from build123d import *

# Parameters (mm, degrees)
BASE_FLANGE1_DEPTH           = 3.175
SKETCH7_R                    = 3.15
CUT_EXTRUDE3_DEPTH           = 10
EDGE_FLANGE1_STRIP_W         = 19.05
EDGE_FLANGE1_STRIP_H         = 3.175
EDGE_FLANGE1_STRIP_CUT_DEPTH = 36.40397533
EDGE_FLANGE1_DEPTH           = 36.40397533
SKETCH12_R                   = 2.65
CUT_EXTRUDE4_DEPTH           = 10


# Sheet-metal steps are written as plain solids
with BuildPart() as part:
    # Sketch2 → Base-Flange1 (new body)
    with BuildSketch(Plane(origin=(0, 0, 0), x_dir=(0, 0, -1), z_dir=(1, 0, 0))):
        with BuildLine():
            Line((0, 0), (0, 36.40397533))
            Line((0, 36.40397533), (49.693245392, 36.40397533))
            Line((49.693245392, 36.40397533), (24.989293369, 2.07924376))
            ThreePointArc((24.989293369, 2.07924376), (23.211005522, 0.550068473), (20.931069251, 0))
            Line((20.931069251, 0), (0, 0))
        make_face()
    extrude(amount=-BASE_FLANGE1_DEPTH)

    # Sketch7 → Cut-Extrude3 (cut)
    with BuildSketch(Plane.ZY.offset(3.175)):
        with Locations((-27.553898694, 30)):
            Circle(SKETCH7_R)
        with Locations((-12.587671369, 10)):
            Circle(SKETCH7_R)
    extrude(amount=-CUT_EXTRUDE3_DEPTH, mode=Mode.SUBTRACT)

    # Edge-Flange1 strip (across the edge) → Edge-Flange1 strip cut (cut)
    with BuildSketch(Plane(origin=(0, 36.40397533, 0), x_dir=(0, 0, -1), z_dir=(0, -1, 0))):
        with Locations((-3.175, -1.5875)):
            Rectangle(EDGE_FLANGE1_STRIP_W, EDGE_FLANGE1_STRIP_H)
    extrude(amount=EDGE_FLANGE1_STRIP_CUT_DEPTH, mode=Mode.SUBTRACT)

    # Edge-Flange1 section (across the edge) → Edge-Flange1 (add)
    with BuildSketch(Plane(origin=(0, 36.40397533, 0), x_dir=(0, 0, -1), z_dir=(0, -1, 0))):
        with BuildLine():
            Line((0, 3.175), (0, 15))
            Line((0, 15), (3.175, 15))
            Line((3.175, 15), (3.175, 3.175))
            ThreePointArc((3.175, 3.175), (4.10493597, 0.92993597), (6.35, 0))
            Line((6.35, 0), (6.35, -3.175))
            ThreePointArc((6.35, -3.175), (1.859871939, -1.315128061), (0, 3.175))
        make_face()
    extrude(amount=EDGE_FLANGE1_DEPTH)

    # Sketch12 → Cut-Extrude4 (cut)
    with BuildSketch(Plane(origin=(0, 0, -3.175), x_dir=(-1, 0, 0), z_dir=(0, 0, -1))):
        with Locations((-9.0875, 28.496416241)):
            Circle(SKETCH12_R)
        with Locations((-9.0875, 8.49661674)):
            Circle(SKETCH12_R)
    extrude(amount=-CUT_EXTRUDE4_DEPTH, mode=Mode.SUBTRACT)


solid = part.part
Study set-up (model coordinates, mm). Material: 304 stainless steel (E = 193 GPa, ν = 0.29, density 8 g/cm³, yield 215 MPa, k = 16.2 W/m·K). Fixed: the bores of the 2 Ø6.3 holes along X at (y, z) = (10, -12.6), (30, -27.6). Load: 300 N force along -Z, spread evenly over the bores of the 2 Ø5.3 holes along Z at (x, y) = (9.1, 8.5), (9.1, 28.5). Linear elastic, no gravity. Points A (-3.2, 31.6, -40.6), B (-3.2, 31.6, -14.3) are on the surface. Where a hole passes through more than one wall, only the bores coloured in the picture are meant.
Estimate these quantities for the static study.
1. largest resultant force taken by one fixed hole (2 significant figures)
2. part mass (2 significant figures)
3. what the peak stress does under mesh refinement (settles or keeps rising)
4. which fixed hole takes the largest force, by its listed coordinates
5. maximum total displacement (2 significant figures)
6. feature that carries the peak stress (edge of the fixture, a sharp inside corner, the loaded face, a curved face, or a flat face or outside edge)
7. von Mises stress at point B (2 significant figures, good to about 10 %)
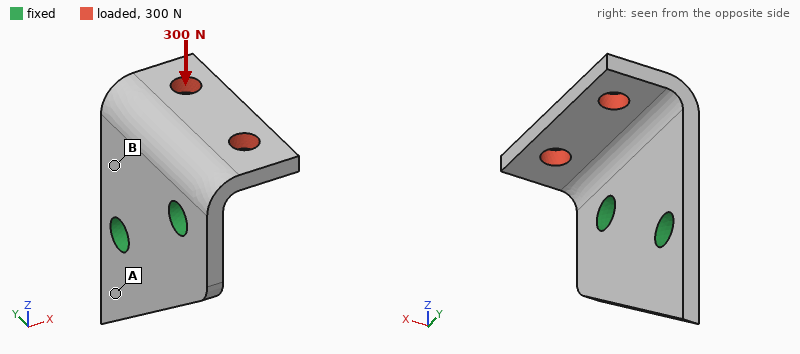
180 N
43 g
keeps rising
(10, -12.6)
45 µm
edge of the fixture
23 MPa
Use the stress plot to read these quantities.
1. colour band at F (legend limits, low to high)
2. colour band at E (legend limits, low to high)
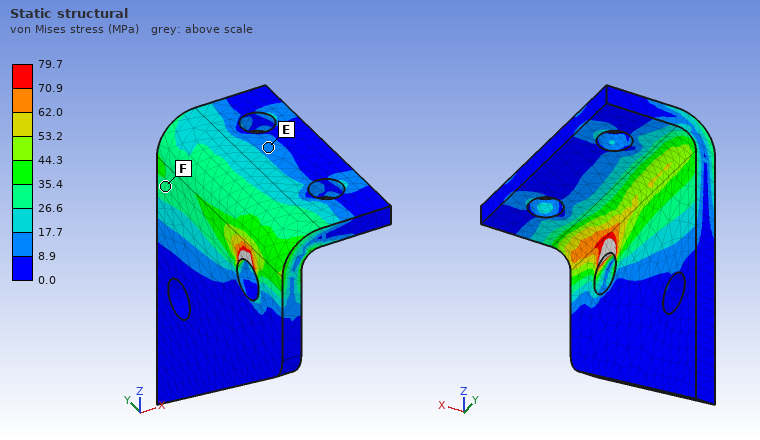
26.6 to 35.4 MPa
8.9 to 17.7 MPa
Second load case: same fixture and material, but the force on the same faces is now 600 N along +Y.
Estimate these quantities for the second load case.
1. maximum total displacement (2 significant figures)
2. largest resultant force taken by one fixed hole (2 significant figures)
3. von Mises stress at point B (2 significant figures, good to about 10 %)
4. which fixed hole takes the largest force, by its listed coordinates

54 µm
640 N
38 MPa
(10, -12.6)
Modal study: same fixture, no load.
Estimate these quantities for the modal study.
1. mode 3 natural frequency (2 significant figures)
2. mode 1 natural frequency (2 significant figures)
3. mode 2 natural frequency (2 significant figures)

10 kHz
4000 Hz
6200 Hz
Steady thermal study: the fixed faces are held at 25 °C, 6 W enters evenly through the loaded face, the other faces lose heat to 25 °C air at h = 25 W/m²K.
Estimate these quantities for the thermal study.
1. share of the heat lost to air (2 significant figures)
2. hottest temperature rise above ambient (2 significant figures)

33 %
66 K
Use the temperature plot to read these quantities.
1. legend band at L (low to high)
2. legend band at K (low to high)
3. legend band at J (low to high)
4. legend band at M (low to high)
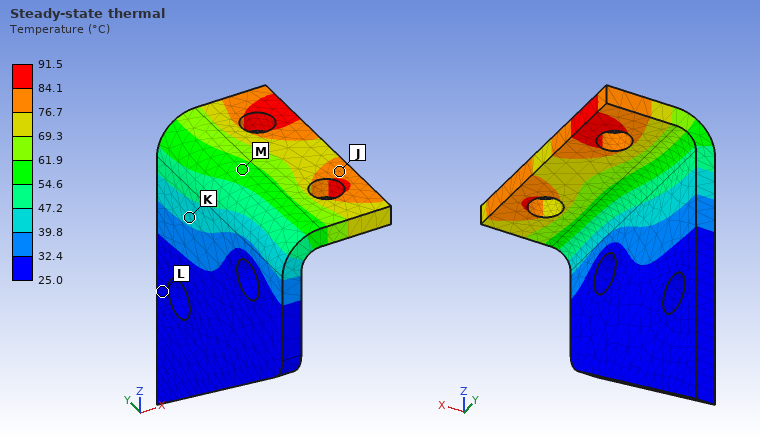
25.0 to 32.4 °C
39.8 to 47.2 °C
76.7 to 84.1 °C
54.6 to 61.9 °C
